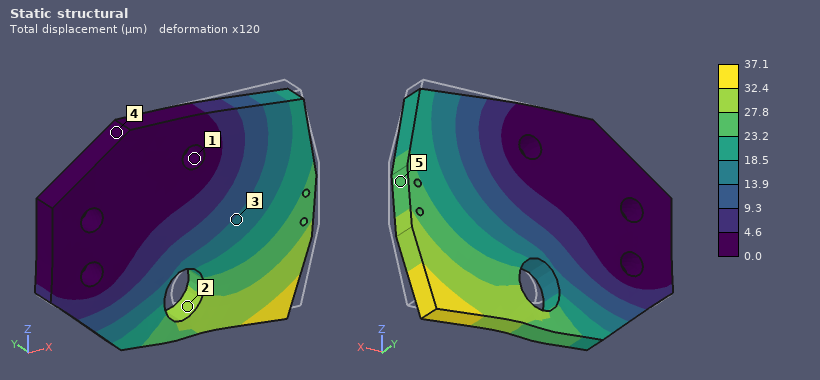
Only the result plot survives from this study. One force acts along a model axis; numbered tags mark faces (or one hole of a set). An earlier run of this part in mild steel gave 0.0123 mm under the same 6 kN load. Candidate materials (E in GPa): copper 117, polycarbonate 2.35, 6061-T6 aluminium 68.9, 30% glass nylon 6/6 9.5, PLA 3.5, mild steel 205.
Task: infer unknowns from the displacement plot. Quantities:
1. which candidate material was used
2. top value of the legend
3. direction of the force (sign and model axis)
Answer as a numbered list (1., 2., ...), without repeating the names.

1. 6061-T6 aluminium
2. 37.1 µm
3. -X
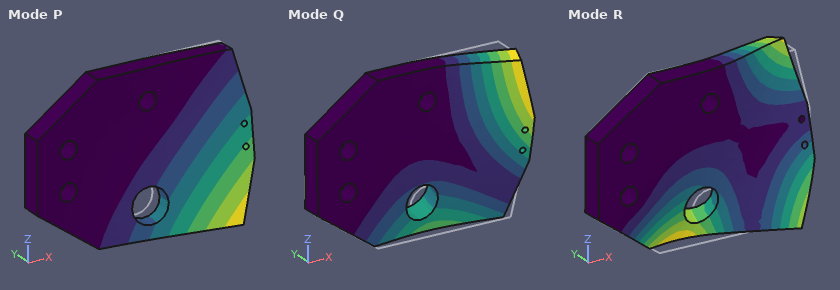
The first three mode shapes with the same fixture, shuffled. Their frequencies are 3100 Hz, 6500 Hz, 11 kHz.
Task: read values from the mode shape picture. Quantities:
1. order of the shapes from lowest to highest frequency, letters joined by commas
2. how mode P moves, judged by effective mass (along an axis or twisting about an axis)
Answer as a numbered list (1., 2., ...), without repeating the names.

1. P, Q, R
2. along Y
